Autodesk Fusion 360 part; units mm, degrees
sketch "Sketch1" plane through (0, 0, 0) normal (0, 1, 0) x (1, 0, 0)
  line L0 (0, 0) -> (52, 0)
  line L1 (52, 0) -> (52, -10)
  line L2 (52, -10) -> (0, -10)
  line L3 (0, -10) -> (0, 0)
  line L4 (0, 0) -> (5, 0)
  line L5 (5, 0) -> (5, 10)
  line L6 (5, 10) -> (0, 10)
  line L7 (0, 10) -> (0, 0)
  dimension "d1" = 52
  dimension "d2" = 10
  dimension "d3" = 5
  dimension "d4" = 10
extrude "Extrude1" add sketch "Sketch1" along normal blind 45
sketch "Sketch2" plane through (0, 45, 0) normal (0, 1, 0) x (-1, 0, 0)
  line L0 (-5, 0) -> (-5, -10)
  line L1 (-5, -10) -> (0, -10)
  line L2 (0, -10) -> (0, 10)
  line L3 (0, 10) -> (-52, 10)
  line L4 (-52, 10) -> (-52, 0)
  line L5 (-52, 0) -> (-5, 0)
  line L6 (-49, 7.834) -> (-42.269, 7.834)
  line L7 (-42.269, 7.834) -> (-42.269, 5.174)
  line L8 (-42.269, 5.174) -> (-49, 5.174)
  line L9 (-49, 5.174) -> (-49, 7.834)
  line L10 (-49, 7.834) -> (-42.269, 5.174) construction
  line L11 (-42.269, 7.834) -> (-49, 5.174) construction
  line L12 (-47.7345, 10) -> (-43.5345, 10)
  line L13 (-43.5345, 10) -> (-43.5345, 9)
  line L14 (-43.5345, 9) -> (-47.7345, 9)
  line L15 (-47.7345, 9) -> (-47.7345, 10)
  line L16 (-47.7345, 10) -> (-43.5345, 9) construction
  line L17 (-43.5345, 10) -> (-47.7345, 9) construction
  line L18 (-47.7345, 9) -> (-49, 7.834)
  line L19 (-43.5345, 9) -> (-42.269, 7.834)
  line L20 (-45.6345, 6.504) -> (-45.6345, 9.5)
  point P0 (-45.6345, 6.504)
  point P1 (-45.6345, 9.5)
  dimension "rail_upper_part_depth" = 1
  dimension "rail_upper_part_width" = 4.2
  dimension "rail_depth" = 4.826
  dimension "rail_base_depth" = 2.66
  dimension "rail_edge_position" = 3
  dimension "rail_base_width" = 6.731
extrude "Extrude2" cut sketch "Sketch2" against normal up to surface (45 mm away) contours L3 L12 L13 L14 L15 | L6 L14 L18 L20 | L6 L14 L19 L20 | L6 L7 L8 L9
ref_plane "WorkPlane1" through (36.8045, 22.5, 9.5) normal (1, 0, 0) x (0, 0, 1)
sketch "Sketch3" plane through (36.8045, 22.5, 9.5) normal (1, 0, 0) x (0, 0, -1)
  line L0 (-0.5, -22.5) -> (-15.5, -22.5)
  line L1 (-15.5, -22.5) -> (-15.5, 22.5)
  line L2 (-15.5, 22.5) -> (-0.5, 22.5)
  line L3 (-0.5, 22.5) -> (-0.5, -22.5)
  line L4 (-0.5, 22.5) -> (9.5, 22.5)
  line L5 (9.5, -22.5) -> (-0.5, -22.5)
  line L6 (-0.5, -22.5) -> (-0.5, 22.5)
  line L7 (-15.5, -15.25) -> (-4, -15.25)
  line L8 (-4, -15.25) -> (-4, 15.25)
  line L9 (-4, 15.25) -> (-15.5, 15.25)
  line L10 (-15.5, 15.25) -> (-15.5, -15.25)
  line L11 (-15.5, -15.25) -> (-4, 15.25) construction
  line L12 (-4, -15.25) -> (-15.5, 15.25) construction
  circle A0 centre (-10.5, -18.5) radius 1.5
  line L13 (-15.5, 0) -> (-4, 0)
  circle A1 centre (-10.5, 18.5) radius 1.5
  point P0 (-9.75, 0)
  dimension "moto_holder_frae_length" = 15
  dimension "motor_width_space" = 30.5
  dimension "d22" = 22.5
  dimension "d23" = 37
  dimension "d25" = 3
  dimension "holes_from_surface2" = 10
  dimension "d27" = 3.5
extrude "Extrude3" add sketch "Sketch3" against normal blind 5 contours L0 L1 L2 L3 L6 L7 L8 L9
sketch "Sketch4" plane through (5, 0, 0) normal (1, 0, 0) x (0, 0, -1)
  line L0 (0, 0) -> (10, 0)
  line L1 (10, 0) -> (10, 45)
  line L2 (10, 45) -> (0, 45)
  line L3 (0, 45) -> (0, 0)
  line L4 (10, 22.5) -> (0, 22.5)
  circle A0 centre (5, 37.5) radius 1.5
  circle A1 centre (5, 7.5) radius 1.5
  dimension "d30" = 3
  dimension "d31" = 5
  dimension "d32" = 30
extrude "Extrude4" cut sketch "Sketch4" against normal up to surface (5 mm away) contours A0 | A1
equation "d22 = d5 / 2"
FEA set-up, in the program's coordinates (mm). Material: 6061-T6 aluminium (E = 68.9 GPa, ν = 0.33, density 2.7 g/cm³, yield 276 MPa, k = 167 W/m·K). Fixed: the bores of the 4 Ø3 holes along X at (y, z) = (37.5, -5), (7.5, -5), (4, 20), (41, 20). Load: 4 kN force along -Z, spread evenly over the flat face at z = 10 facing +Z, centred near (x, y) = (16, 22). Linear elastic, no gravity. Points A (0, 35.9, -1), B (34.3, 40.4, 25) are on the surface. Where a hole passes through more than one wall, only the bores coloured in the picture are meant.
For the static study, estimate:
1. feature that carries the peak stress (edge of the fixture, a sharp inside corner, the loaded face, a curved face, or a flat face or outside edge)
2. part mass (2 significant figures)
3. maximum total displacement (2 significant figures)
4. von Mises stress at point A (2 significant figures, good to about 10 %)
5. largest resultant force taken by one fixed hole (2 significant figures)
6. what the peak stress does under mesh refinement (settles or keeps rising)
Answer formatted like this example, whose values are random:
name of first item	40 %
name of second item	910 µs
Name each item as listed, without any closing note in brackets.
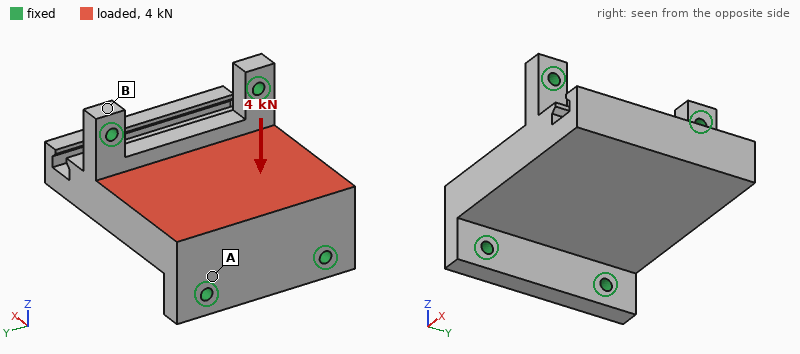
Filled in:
feature that carries the peak stress	edge of the fixture
part mass	70 g
maximum total displacement	12 µm
von Mises stress at point A	14 MPa
largest resultant force taken by one fixed hole	1.2 kN
what the peak stress does under mesh refinement	keeps rising
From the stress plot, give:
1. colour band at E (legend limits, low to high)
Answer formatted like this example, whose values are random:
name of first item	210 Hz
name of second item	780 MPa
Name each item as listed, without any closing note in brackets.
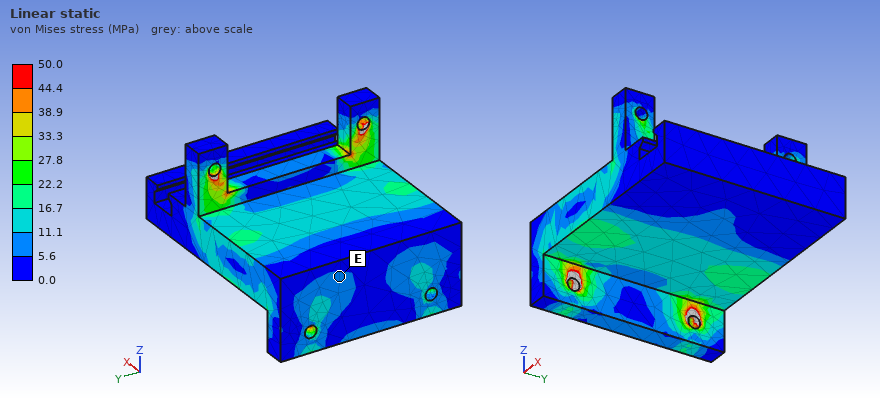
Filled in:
colour band at E	5.6 to 11.1 MPa
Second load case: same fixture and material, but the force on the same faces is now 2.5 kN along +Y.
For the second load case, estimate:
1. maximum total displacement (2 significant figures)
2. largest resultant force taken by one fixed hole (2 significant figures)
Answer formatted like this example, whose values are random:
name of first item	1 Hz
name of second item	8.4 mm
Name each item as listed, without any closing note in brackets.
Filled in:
maximum total displacement	9.0 µm
largest resultant force taken by one fixed hole	1.1 kN
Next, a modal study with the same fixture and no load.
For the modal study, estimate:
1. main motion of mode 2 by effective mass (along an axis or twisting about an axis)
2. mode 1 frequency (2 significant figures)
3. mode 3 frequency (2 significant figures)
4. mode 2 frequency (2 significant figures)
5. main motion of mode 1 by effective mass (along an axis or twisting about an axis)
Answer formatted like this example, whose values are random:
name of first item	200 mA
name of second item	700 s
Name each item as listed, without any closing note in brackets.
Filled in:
main motion of mode 2 by effective mass	along X
mode 1 frequency	8300 Hz
mode 3 frequency	11 kHz
mode 2 frequency	8800 Hz
main motion of mode 1 by effective mass	along Y
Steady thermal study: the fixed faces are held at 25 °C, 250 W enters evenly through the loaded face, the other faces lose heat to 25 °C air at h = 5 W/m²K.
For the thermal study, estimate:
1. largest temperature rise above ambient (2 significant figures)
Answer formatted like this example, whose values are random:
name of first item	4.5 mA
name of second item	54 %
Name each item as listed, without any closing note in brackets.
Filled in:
largest temperature rise above ambient	75 K
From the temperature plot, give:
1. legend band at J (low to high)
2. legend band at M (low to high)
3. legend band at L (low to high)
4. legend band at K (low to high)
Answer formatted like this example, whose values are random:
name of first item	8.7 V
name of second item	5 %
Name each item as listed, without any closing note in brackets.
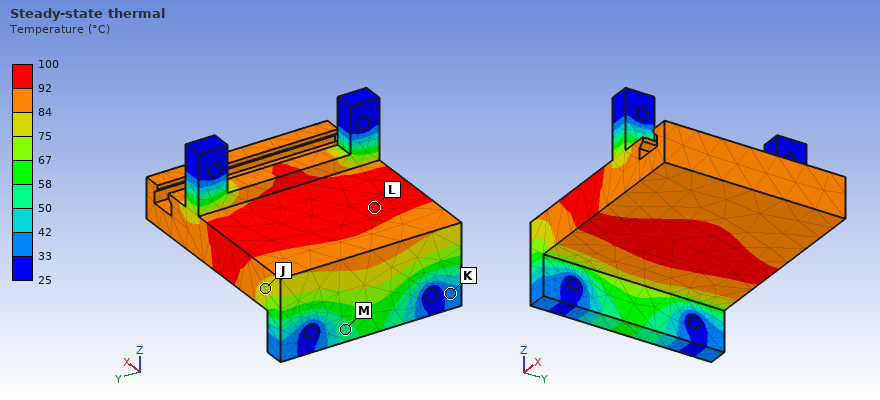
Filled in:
legend band at J	75 to 84 °C
legend band at M	50 to 58 °C
legend band at L	92 to 100 °C
legend band at K	33 to 42 °C
